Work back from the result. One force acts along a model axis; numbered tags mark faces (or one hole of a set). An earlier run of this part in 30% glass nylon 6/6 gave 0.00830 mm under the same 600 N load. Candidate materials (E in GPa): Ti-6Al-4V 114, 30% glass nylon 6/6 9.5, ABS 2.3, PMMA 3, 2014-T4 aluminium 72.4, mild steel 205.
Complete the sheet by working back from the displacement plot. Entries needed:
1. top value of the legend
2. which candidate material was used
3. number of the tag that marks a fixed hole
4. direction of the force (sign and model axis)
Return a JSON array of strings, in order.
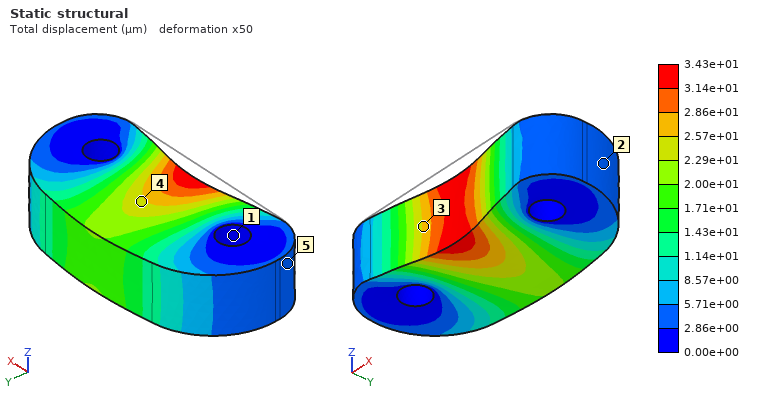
["3.43e+01 µm", "ABS", "1", "+Y"]
